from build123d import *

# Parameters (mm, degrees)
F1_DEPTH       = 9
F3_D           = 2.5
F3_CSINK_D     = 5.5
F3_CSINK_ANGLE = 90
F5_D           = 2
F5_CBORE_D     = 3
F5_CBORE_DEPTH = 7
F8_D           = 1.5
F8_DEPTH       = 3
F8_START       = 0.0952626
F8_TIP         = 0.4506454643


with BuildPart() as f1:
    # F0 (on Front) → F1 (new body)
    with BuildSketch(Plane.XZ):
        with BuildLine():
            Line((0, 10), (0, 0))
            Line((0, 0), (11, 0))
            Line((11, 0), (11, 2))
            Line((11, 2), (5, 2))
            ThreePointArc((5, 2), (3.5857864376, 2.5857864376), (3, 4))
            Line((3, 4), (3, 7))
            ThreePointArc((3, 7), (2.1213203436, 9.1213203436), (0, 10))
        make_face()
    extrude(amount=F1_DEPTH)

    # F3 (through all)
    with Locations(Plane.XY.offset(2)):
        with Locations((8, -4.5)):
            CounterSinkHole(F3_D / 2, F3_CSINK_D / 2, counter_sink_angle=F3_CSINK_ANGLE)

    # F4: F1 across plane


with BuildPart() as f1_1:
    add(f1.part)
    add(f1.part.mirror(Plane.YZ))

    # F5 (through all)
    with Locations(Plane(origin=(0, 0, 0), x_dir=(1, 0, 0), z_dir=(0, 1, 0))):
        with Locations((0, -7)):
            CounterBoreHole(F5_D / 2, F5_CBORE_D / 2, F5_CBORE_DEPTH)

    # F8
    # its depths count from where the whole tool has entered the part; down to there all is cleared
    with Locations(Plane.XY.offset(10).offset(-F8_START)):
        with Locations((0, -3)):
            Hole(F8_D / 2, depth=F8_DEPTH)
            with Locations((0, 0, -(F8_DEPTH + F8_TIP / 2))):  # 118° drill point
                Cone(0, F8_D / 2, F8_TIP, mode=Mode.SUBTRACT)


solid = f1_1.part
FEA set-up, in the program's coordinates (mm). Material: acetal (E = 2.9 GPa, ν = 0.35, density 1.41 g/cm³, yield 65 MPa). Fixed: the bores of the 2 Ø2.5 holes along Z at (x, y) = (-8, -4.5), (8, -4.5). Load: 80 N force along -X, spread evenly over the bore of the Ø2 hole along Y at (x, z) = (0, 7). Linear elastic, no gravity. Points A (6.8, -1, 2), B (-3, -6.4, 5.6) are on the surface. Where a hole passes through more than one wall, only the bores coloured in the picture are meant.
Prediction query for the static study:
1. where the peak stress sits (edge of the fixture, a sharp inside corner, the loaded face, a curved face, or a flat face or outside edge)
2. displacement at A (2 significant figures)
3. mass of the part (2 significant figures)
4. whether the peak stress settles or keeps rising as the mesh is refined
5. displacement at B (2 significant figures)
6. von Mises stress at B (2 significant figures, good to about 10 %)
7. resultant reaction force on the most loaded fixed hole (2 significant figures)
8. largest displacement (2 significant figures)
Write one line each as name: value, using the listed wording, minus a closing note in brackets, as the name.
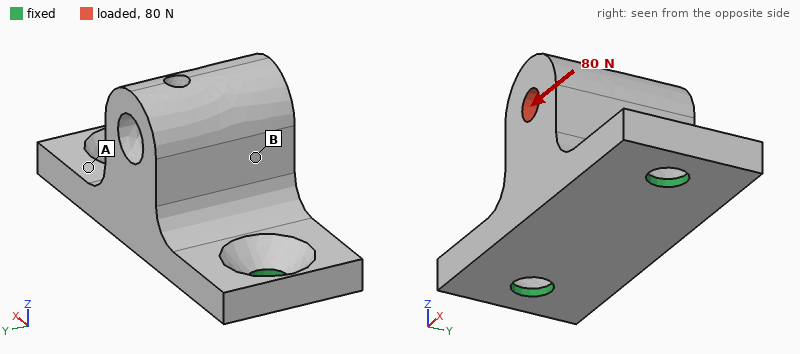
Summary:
where the peak stress sits: edge of the fixture
displacement at A: 0.022 mm
mass of the part: 1.00 g
whether the peak stress settles or keeps rising as the mesh is refined: keeps rising
displacement at B: 0.058 mm
von Mises stress at B: 7.0 MPa
resultant reaction force on the most loaded fixed hole: 58 N
largest displacement: 0.11 mm
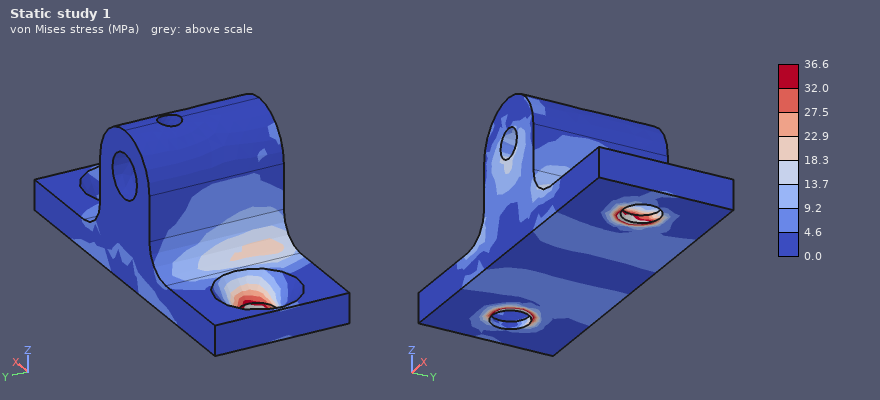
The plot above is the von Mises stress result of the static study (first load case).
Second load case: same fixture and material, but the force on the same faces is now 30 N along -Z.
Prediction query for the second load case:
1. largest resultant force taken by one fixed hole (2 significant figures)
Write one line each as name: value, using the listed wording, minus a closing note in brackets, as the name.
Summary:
largest resultant force taken by one fixed hole: 24 N
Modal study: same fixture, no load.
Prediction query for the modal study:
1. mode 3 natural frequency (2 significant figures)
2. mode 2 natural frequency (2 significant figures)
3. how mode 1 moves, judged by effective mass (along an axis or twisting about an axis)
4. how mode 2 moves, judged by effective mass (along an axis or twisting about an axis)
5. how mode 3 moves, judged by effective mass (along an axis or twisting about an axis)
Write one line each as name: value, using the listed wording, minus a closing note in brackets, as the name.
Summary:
mode 3 natural frequency: 9100 Hz
mode 2 natural frequency: 7200 Hz
how mode 1 moves, judged by effective mass: along Y
how mode 2 moves, judged by effective mass: along Z
how mode 3 moves, judged by effective mass: along X
